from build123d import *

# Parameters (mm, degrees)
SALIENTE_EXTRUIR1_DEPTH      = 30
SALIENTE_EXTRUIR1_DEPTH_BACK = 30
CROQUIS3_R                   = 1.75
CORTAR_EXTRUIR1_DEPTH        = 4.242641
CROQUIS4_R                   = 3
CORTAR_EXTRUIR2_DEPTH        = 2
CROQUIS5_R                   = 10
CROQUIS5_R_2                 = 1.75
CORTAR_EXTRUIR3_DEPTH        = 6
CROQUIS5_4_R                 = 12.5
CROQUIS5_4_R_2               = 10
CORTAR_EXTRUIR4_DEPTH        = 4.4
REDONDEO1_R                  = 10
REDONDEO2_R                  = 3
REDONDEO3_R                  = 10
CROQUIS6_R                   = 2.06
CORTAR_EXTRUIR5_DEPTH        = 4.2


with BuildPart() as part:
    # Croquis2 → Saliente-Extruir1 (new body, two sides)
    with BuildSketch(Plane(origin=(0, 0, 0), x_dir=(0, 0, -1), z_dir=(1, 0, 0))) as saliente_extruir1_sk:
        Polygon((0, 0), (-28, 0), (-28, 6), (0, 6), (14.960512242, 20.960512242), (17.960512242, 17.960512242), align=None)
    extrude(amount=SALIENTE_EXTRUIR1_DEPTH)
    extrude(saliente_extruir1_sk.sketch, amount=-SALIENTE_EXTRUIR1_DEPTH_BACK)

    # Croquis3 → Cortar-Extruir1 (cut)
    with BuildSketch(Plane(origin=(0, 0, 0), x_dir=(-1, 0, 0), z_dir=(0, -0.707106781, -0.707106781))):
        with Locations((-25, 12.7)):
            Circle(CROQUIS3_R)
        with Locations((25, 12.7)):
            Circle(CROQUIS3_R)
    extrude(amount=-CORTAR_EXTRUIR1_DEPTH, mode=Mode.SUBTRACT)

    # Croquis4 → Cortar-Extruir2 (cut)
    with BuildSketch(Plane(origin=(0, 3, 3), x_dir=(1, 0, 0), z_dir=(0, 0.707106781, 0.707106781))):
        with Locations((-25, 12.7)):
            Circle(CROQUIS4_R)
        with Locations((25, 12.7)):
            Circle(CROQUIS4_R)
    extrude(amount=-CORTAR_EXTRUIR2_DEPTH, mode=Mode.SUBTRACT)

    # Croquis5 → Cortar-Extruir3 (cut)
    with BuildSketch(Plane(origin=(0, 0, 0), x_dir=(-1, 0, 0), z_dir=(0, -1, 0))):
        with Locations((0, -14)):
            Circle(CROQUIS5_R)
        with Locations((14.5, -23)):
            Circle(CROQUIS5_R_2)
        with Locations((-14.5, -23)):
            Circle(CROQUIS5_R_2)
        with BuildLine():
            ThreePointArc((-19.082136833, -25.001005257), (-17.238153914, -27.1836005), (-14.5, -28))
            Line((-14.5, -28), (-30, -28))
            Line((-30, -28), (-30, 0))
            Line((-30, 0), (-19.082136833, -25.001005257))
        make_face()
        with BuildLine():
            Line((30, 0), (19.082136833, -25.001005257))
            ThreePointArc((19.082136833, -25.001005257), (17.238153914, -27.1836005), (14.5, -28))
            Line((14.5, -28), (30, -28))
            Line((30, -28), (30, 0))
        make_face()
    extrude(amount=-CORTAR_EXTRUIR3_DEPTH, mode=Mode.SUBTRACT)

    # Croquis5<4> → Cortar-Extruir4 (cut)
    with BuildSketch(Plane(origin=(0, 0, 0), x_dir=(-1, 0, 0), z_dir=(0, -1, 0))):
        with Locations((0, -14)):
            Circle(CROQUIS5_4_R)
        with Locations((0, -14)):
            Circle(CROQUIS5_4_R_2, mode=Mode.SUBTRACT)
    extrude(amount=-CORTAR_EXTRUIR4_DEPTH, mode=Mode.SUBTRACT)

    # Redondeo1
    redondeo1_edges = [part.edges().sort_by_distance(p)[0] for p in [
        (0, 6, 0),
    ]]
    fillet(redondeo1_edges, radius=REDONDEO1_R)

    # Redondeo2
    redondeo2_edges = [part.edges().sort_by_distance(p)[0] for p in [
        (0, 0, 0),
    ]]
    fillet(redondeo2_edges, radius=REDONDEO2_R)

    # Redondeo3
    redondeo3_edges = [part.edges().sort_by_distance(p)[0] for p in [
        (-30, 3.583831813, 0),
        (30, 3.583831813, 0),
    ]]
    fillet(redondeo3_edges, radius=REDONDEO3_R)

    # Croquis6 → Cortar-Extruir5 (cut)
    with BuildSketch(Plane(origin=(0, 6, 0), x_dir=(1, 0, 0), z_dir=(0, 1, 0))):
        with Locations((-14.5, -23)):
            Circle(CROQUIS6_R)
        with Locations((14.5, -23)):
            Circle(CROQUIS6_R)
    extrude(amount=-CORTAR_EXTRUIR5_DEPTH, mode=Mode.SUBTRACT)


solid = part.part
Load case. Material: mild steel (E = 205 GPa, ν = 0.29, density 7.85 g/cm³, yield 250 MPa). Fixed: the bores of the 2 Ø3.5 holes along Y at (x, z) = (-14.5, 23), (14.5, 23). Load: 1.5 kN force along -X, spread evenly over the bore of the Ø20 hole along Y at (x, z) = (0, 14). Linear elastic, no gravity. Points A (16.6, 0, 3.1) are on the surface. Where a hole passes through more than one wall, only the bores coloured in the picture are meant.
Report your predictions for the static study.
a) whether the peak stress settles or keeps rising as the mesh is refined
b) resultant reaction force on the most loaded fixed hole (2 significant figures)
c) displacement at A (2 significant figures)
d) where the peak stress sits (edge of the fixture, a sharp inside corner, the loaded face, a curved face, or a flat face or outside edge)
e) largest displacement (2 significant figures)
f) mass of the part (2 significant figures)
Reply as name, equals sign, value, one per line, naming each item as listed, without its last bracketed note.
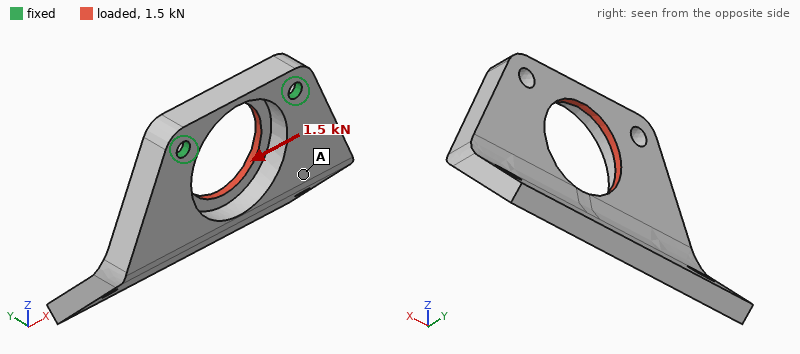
whether the peak stress settles or keeps rising as the mesh is refined = keeps rising
resultant reaction force on the most loaded fixed hole = 840 N
displacement at A = 7.2 µm
where the peak stress sits = edge of the fixture
largest displacement = 12 µm
mass of the part = 87 g
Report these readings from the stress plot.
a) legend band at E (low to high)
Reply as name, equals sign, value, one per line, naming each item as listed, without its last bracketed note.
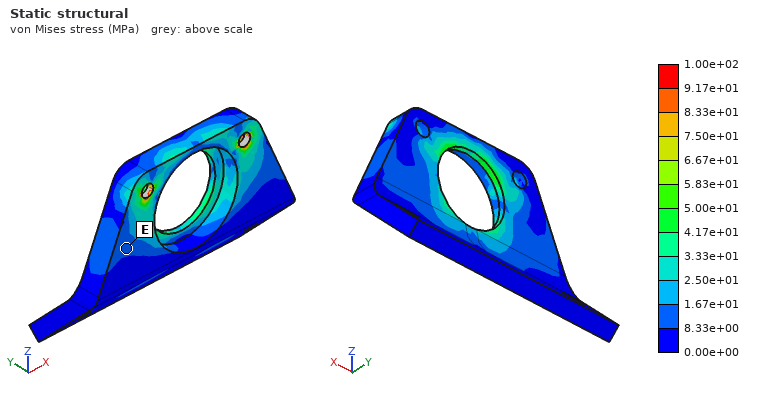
legend band at E = 8.33e+00 to 1.67e+01 MPa
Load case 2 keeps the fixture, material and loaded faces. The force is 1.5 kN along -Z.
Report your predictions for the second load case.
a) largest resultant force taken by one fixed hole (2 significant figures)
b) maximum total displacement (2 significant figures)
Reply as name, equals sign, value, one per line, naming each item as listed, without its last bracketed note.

largest resultant force taken by one fixed hole = 750 N
maximum total displacement = 58 µm
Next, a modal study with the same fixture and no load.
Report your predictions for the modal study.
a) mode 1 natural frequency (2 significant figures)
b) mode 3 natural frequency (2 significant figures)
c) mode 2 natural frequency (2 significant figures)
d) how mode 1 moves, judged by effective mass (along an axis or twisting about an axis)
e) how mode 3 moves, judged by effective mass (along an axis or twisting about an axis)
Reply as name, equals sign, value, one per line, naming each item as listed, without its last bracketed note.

mode 1 natural frequency = 1300 Hz
mode 3 natural frequency = 5000 Hz
mode 2 natural frequency = 2800 Hz
how mode 1 moves, judged by effective mass = along Y
how mode 3 moves, judged by effective mass = along X
